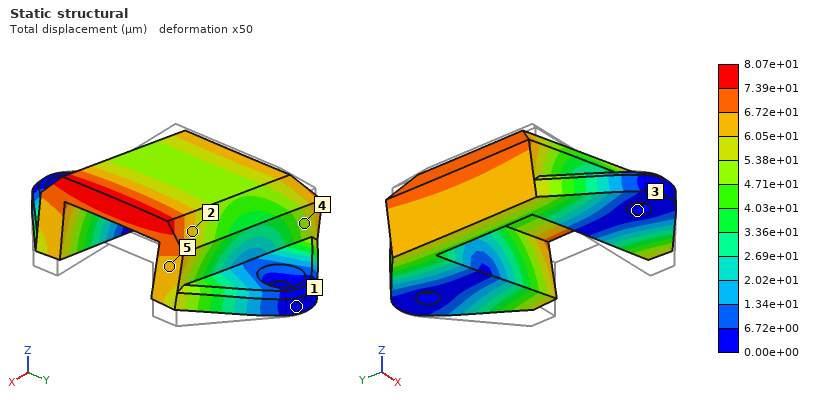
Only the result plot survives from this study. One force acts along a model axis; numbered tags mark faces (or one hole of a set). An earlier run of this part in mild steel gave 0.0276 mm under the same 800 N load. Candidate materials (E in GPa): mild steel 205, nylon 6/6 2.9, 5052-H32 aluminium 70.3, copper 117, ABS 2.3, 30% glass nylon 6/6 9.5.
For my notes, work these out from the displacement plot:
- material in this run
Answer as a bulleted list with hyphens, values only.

- 5052-H32 aluminium
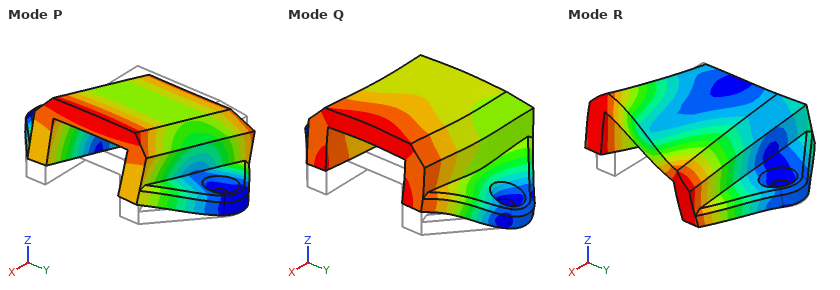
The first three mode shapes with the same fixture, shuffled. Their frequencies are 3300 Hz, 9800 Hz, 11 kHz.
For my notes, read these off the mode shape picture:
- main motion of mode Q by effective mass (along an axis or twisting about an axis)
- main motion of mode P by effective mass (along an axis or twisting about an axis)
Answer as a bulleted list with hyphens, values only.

- along Z
- along X
